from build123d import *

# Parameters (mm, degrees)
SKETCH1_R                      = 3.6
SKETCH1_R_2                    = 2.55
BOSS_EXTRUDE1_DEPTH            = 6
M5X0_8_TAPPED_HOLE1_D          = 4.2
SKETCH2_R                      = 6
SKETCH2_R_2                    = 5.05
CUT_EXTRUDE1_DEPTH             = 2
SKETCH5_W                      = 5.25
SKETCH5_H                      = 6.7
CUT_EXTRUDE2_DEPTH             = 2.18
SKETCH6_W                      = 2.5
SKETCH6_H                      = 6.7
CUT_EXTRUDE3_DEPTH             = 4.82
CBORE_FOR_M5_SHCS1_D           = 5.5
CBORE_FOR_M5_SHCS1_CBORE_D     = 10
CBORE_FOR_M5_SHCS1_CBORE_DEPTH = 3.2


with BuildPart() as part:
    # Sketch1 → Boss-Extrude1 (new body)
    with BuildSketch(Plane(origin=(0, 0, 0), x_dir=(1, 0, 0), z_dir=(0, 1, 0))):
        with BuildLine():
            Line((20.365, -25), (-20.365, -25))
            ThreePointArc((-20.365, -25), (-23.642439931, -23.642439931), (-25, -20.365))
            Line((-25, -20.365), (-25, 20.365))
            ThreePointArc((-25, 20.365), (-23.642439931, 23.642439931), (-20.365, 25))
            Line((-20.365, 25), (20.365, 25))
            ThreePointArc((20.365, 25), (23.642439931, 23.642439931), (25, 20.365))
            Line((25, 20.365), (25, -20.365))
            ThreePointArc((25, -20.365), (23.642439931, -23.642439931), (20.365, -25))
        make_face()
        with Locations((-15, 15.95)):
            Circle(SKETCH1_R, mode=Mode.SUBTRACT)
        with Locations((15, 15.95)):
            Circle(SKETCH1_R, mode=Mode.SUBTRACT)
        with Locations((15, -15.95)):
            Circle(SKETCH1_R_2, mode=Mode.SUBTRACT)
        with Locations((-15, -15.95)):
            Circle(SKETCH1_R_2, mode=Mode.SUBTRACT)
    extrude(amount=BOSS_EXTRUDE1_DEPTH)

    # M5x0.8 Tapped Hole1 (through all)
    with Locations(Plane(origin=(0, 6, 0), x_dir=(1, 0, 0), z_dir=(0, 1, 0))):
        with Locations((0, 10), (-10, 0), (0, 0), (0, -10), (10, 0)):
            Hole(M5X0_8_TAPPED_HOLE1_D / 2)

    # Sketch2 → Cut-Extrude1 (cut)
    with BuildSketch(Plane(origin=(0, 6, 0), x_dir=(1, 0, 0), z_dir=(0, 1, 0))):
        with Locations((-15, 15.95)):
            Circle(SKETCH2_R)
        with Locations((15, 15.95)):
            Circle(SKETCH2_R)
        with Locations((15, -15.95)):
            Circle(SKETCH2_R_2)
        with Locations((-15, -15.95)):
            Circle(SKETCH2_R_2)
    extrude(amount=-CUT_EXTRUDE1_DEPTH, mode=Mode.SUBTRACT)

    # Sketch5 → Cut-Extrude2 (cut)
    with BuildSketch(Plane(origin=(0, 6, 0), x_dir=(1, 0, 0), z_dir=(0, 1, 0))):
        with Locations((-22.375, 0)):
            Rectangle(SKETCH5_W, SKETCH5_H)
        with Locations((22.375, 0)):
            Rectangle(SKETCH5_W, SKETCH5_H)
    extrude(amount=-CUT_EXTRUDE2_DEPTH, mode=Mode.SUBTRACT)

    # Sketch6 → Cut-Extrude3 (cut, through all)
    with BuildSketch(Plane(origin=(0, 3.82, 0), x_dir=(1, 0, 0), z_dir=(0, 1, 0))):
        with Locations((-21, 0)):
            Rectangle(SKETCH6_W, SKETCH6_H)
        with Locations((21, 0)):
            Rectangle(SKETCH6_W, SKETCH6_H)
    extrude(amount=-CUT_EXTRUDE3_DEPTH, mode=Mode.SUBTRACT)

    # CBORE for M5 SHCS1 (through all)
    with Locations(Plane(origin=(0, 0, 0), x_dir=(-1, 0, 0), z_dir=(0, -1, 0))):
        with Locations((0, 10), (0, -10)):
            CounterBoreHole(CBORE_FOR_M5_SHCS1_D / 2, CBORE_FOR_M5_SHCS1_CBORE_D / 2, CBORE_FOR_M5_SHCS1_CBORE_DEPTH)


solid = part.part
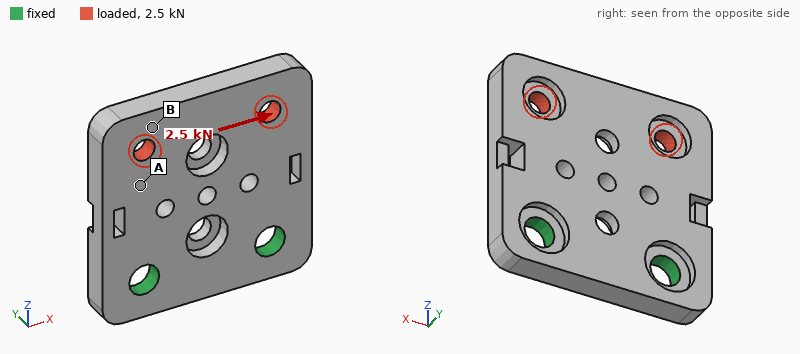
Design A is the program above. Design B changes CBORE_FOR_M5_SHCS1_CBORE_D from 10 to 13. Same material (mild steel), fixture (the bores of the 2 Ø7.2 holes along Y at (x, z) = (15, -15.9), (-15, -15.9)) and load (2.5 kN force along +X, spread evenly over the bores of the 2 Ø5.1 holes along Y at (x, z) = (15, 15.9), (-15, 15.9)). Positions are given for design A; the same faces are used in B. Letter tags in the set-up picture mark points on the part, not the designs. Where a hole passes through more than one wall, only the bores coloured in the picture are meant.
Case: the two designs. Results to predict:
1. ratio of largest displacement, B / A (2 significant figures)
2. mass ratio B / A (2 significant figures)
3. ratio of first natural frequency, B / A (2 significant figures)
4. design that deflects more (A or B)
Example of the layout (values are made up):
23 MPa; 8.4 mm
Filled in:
1.2; 0.97; 0.99; B
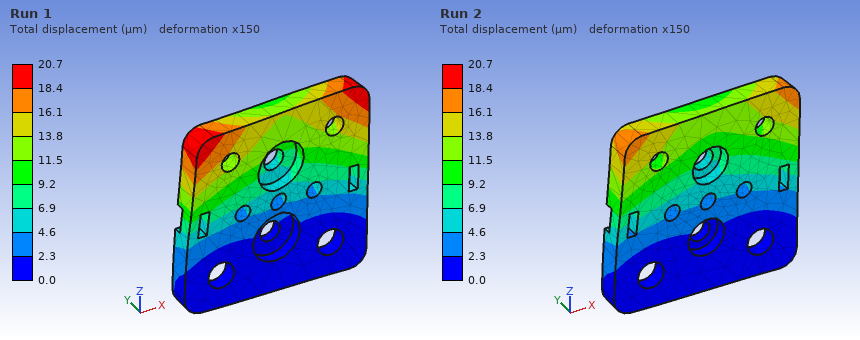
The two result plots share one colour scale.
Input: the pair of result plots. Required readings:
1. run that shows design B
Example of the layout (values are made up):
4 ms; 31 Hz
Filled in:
Run 1
